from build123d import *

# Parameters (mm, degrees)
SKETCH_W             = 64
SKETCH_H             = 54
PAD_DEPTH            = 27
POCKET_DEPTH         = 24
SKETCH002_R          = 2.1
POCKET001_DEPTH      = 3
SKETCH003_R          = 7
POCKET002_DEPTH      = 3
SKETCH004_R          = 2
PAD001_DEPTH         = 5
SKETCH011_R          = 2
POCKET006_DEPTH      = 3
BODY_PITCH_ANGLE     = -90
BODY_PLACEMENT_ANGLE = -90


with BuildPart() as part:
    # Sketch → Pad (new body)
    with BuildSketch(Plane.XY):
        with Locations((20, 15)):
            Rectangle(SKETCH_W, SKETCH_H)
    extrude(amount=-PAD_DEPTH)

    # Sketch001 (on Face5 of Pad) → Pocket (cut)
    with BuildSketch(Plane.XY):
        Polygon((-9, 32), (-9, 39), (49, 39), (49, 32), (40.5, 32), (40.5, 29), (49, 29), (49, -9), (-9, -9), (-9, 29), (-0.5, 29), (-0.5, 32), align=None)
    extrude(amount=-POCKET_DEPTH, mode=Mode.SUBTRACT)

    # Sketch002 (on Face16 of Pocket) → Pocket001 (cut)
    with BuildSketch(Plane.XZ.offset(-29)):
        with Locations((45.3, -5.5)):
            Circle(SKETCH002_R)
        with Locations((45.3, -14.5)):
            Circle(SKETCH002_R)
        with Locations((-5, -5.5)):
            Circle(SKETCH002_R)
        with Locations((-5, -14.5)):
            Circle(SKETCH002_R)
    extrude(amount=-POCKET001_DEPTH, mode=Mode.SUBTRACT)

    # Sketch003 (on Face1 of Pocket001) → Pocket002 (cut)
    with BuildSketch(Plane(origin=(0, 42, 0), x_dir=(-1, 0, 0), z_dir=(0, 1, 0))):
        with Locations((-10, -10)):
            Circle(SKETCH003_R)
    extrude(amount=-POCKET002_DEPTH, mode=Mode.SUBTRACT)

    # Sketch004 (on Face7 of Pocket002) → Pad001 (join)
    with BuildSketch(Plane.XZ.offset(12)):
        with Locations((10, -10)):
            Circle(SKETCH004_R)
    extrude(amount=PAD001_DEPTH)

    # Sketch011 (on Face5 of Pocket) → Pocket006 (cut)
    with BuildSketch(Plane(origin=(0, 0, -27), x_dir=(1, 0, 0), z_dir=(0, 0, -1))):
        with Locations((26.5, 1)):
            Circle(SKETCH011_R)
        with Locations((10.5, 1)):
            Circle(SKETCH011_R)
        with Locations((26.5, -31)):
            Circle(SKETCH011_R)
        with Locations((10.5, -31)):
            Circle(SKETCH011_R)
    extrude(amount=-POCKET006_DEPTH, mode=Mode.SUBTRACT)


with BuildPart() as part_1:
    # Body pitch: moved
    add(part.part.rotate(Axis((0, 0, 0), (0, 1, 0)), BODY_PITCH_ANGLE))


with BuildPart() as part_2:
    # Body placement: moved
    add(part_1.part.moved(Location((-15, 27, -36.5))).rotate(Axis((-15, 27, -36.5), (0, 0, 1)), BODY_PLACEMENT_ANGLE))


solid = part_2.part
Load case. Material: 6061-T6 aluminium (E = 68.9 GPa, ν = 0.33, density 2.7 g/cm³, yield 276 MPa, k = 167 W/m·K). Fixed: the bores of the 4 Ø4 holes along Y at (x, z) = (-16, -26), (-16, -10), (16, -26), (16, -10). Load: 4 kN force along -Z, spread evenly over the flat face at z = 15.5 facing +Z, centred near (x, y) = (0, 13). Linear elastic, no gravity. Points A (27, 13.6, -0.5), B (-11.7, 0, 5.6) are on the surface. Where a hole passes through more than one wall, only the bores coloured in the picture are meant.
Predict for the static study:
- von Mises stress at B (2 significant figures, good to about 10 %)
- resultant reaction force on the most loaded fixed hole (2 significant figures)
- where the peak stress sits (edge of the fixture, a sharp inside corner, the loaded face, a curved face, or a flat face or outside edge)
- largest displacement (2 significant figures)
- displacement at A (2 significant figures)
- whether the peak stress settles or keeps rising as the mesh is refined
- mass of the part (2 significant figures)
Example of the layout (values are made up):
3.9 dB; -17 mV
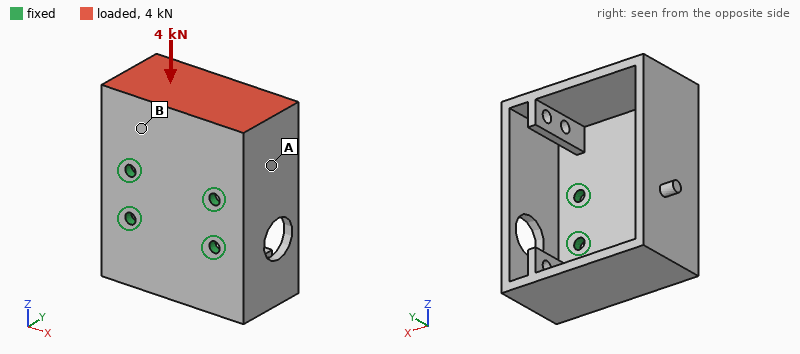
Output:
37 MPa; 1.7 kN; edge of the fixture; 0.49 mm; 0.10 mm; keeps rising; 73 g
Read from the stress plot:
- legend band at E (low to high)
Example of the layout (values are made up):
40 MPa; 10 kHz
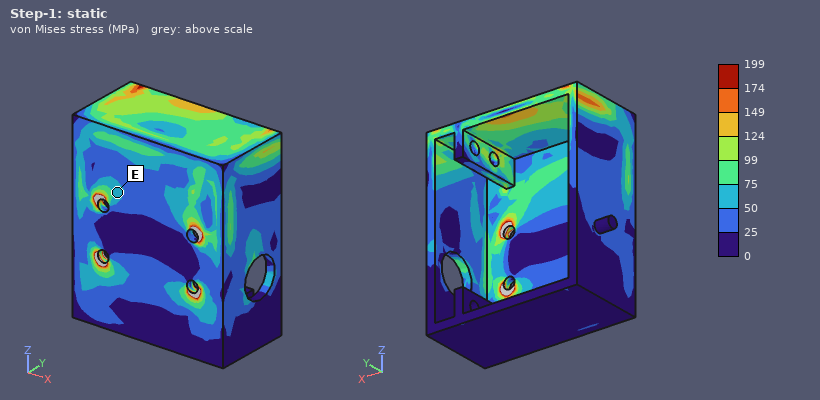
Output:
50 to 75 MPa
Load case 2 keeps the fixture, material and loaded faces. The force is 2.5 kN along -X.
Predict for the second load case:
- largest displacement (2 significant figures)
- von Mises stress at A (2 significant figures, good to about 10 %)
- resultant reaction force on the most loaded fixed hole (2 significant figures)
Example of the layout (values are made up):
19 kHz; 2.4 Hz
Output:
0.24 mm; 29 MPa; 2.1 kN
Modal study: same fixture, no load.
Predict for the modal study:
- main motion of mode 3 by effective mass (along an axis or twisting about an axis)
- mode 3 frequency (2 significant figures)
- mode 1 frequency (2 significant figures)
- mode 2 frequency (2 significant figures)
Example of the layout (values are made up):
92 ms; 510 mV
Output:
along X; 3900 Hz; 2600 Hz; 2800 Hz
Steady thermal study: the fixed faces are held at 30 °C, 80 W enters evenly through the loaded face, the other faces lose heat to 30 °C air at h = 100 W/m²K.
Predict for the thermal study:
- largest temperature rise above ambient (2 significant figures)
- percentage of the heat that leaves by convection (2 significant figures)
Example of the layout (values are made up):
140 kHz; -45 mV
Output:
56 K; 32 %
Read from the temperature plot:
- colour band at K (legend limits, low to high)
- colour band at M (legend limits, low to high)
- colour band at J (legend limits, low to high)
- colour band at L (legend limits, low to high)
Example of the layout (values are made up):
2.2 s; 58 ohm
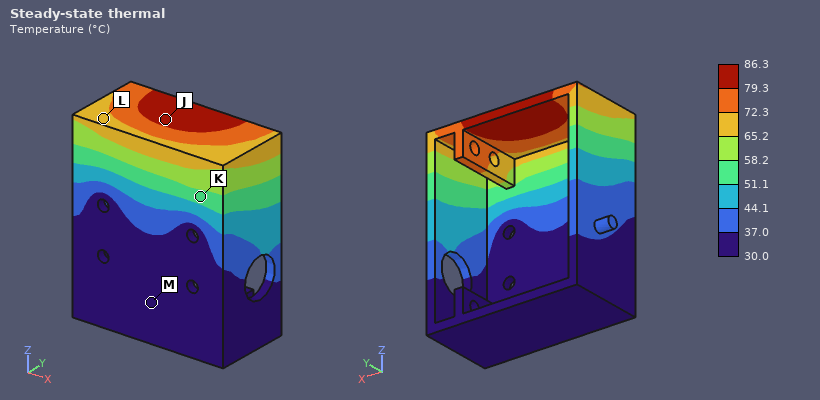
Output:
51.1 to 58.2 °C; 30.0 to 37.0 °C; 79.3 to 86.3 °C; 65.2 to 72.3 °C
